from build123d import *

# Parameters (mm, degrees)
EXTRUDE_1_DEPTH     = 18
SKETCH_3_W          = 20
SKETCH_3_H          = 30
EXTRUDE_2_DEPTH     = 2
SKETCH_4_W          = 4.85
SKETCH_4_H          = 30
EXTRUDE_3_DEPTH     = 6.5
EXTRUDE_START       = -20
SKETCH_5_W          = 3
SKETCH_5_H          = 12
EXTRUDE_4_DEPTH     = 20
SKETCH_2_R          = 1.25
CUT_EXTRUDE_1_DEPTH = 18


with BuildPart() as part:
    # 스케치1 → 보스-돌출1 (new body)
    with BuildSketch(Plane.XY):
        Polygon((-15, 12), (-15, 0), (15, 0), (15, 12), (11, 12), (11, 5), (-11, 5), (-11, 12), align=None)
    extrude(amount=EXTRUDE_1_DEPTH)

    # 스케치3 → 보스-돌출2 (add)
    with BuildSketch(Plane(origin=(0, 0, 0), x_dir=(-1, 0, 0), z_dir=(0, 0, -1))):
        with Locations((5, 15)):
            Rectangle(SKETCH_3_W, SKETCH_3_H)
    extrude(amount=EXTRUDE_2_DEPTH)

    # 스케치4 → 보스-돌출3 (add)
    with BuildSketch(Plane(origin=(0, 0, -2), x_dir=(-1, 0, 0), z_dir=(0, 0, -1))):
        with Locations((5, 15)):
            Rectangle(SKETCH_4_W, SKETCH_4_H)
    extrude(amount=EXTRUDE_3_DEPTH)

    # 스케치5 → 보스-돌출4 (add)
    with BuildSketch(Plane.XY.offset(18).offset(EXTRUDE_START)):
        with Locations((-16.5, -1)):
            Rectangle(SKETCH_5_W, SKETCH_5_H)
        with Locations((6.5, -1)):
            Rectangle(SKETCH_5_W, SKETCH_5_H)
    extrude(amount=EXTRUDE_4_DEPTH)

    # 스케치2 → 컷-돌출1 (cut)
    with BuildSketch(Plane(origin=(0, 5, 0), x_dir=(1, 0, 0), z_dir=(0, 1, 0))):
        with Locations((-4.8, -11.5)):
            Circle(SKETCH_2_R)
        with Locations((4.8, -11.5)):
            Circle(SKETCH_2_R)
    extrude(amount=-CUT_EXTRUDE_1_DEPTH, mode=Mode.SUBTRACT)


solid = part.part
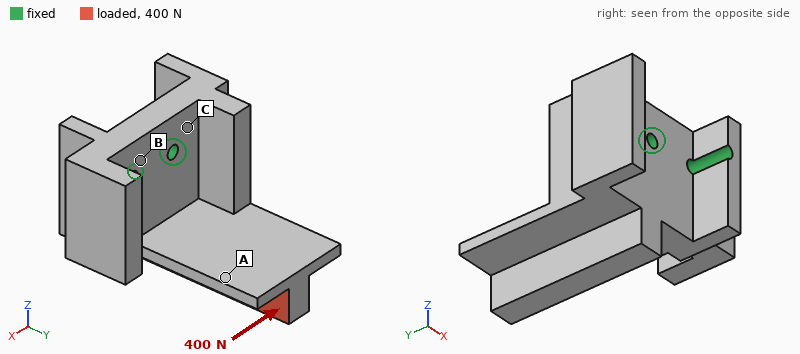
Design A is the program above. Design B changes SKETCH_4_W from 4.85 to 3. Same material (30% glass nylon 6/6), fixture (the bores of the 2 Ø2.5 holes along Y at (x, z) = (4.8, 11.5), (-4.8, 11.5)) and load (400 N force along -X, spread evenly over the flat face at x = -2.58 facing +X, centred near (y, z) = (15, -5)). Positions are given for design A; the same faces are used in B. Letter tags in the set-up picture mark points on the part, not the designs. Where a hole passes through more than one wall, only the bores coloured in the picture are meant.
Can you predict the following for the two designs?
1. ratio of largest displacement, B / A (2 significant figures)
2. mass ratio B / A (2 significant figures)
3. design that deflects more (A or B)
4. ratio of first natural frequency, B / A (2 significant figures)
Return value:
1.3
0.95
B
1.0
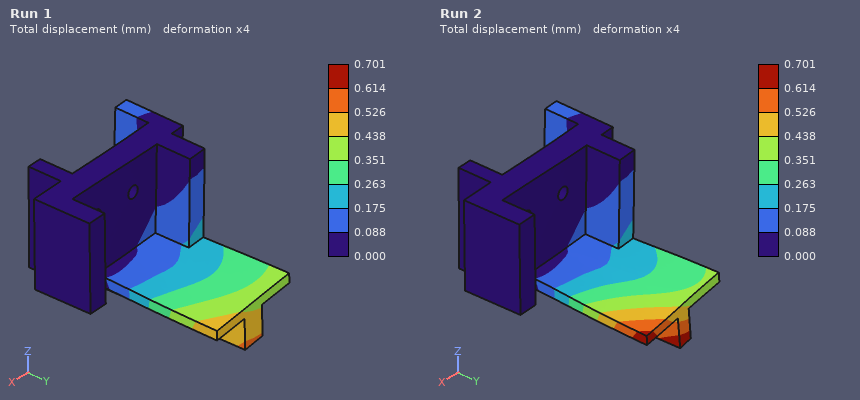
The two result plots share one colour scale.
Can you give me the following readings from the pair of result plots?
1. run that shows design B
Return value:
Run 2
